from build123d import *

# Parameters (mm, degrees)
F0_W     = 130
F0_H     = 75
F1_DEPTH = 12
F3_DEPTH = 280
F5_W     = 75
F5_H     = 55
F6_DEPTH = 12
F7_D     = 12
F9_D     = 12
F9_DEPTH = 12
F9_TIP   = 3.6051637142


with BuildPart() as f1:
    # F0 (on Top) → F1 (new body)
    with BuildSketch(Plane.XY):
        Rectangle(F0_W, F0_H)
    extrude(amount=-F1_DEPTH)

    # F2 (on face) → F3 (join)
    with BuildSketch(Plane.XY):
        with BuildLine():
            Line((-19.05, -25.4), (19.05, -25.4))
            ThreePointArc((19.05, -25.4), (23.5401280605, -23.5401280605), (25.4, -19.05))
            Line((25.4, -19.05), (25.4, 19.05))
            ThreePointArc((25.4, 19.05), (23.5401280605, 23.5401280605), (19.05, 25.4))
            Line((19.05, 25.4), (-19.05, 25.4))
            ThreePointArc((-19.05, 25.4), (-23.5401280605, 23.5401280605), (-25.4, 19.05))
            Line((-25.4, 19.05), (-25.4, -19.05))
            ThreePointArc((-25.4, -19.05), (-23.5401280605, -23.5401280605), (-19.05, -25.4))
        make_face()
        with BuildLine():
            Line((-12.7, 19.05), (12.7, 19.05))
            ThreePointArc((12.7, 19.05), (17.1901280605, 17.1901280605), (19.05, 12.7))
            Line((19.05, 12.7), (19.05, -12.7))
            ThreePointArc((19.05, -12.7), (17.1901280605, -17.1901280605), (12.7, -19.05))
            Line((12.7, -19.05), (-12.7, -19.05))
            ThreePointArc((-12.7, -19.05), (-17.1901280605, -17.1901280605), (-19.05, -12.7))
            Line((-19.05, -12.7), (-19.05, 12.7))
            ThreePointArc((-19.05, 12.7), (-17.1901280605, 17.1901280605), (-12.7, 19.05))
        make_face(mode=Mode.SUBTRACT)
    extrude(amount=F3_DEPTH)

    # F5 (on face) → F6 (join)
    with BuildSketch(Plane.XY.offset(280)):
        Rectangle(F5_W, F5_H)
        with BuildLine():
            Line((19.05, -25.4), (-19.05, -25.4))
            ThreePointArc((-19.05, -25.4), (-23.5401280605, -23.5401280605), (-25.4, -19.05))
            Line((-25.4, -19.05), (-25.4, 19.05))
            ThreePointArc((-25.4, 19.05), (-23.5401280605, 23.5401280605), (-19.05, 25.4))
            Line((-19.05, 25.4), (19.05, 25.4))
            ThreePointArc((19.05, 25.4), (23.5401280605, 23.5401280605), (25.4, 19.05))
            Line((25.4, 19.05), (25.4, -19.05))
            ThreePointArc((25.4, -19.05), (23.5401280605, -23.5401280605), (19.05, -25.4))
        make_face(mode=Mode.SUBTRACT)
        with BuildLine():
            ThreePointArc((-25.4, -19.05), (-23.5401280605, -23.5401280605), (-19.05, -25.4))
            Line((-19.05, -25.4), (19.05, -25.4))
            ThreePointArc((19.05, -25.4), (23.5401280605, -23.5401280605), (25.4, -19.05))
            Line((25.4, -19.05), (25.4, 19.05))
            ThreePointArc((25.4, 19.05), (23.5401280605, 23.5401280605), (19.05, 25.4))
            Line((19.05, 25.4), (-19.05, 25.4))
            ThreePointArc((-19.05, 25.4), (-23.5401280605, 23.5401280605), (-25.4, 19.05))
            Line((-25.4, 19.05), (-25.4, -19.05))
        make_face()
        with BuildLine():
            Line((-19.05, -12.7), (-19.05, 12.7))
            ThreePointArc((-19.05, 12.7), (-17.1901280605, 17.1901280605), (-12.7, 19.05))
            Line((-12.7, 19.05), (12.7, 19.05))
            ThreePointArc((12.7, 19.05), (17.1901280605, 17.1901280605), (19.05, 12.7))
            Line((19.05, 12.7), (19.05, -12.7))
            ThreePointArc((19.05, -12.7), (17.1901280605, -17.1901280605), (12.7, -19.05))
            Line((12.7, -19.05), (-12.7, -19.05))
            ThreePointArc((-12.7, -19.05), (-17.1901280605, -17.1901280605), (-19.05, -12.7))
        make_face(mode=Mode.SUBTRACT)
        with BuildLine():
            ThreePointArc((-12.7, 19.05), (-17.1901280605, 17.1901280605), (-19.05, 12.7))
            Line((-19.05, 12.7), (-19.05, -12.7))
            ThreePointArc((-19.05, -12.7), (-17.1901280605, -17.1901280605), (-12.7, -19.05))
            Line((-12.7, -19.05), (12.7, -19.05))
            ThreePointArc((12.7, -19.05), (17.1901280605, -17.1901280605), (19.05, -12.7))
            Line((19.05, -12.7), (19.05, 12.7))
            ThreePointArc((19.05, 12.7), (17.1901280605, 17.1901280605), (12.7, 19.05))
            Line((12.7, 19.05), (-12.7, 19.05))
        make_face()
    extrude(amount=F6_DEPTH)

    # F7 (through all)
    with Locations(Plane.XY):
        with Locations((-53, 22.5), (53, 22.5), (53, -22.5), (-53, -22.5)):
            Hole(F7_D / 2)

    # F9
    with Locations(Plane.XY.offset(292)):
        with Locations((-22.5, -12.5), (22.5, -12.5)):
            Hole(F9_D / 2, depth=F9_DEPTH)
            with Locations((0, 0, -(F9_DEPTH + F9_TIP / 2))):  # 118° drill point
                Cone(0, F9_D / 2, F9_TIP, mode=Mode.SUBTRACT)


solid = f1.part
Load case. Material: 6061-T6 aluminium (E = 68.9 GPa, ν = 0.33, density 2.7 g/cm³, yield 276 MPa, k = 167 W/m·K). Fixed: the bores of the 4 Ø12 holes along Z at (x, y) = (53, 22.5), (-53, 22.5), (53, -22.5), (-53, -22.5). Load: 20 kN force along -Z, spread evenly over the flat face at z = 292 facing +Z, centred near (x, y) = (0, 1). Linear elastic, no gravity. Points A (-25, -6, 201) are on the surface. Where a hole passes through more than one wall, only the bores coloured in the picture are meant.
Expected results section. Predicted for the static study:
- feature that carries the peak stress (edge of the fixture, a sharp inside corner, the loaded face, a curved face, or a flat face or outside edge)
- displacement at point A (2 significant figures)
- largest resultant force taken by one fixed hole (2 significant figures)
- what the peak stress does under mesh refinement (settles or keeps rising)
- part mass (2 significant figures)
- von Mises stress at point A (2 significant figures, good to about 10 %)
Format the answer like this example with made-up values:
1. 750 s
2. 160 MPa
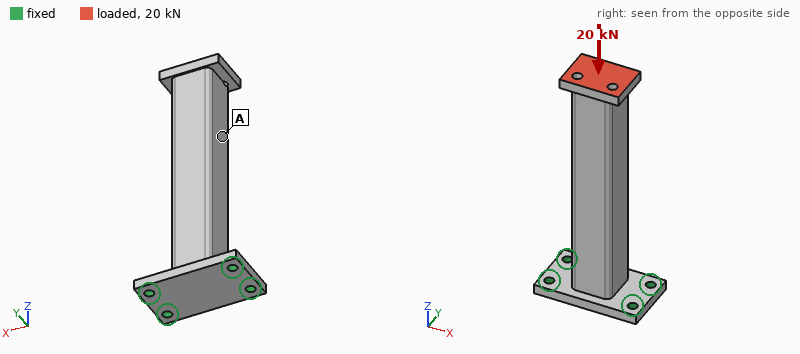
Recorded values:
1. edge of the fixture
2. 0.12 mm
3. 5.3 kN
4. keeps rising
5. 1.3 kg
6. 17 MPa
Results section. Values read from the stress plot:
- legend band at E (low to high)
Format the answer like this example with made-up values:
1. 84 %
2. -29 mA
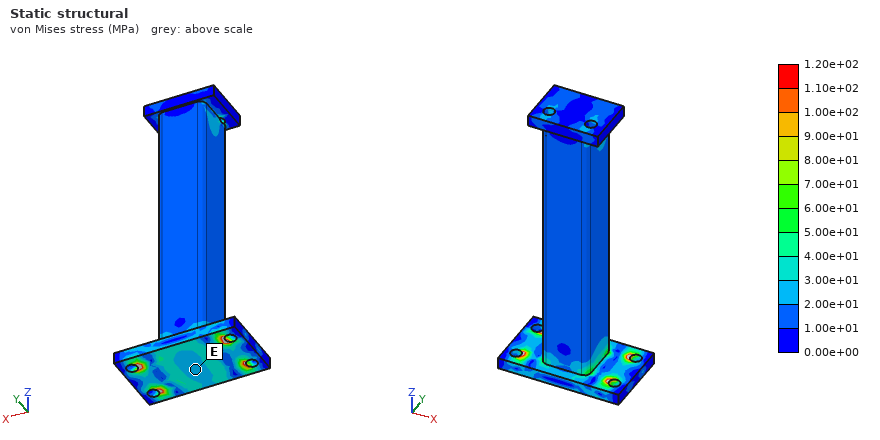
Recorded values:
1. 2.00e+01 to 3.00e+01 MPa
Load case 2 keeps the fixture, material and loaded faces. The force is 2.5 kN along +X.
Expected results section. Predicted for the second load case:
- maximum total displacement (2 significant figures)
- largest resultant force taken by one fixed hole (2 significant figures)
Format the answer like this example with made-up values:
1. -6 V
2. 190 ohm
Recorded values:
1. 1.3 mm
2. 4.9 kN
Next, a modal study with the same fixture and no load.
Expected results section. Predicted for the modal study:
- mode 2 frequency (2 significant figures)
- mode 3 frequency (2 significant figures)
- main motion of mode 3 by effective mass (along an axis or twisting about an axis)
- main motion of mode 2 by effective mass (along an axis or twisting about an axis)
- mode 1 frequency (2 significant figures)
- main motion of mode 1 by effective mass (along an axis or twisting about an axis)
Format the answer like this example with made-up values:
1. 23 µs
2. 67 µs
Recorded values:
1. 380 Hz
2. 2100 Hz
3. twisting about Z
4. along X
5. 300 Hz
6. along Y
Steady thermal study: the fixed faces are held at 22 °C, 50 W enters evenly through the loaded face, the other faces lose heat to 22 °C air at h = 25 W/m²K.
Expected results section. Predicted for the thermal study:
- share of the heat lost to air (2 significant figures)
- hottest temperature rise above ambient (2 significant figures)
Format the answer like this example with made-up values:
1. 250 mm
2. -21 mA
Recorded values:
1. 77 %
2. 36 K
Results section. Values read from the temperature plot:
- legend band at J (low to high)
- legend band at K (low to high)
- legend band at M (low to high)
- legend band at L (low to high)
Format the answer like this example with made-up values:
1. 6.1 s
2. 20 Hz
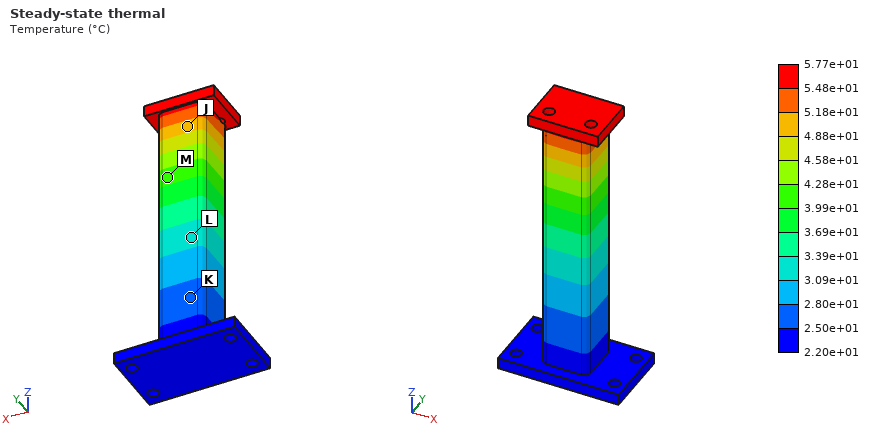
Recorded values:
1. 4.88e+01 to 5.18e+01 °C
2. 2.50e+01 to 2.80e+01 °C
3. 3.99e+01 to 4.28e+01 °C
4. 3.09e+01 to 3.39e+01 °C
